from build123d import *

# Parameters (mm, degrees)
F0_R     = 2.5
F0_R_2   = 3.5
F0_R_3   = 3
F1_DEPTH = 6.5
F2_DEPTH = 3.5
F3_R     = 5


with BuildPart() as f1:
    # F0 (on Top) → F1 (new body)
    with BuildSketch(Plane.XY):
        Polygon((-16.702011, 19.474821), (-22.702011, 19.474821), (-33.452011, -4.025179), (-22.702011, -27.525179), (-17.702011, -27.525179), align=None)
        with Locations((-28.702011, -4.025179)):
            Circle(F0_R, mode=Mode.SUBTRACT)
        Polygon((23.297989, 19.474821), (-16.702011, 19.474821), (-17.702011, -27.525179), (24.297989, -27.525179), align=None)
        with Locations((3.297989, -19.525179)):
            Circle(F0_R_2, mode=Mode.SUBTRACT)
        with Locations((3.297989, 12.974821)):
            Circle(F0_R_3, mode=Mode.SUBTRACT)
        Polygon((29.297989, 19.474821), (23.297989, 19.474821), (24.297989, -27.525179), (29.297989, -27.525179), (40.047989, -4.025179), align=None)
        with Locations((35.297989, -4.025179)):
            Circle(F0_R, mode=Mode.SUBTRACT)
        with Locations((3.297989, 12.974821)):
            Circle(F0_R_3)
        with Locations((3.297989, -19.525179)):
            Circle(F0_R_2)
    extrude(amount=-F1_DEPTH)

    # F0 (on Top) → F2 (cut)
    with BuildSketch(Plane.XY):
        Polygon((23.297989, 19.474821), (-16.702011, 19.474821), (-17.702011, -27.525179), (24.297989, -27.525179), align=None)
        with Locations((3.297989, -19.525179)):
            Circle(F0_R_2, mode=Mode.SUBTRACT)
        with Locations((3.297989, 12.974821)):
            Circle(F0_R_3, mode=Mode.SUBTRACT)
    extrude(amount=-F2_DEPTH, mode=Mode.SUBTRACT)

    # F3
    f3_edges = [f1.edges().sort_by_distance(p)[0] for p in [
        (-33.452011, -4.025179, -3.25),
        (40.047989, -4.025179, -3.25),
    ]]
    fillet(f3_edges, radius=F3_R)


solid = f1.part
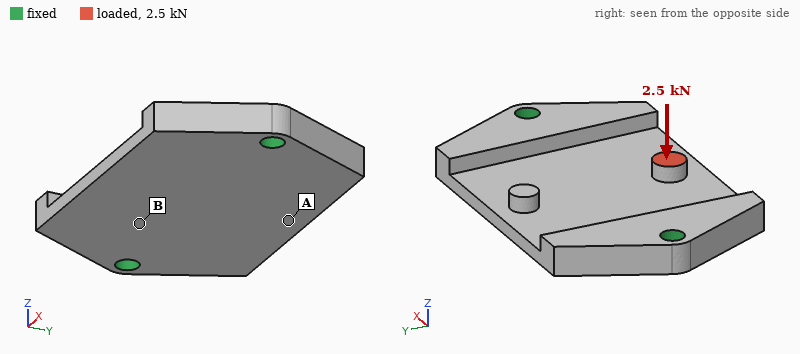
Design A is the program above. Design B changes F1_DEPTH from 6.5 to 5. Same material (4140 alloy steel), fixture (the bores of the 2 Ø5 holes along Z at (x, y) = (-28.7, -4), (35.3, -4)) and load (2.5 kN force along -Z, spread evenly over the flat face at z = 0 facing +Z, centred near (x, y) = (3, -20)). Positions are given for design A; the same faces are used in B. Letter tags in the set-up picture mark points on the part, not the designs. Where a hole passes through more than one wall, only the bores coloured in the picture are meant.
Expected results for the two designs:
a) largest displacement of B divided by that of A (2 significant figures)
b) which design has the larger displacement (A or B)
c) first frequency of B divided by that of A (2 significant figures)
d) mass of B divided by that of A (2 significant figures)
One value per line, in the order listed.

4.6
B
0.70
0.65
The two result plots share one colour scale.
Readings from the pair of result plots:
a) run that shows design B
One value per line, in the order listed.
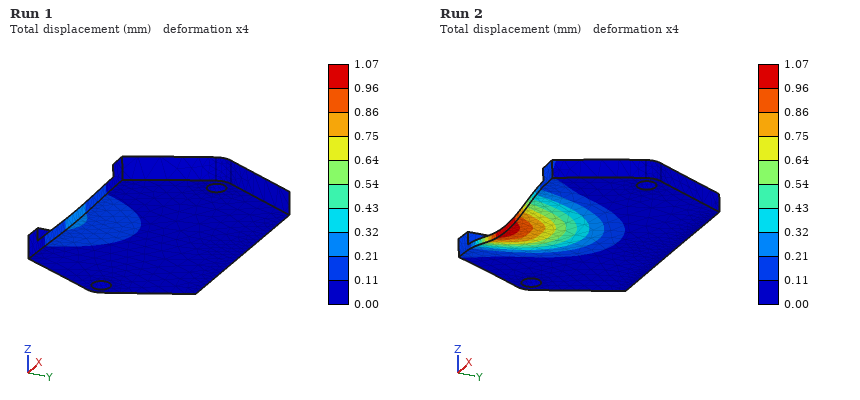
Run 2
